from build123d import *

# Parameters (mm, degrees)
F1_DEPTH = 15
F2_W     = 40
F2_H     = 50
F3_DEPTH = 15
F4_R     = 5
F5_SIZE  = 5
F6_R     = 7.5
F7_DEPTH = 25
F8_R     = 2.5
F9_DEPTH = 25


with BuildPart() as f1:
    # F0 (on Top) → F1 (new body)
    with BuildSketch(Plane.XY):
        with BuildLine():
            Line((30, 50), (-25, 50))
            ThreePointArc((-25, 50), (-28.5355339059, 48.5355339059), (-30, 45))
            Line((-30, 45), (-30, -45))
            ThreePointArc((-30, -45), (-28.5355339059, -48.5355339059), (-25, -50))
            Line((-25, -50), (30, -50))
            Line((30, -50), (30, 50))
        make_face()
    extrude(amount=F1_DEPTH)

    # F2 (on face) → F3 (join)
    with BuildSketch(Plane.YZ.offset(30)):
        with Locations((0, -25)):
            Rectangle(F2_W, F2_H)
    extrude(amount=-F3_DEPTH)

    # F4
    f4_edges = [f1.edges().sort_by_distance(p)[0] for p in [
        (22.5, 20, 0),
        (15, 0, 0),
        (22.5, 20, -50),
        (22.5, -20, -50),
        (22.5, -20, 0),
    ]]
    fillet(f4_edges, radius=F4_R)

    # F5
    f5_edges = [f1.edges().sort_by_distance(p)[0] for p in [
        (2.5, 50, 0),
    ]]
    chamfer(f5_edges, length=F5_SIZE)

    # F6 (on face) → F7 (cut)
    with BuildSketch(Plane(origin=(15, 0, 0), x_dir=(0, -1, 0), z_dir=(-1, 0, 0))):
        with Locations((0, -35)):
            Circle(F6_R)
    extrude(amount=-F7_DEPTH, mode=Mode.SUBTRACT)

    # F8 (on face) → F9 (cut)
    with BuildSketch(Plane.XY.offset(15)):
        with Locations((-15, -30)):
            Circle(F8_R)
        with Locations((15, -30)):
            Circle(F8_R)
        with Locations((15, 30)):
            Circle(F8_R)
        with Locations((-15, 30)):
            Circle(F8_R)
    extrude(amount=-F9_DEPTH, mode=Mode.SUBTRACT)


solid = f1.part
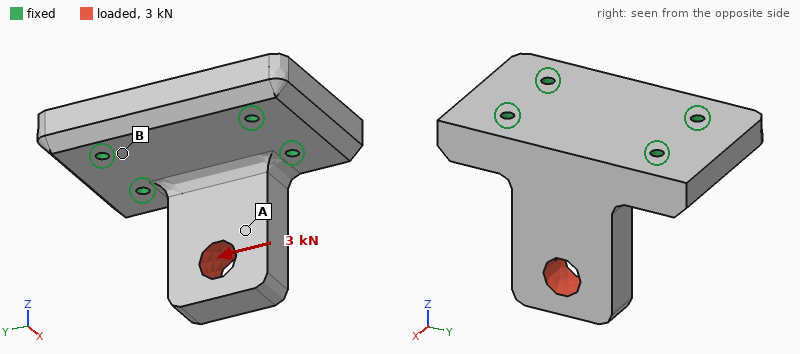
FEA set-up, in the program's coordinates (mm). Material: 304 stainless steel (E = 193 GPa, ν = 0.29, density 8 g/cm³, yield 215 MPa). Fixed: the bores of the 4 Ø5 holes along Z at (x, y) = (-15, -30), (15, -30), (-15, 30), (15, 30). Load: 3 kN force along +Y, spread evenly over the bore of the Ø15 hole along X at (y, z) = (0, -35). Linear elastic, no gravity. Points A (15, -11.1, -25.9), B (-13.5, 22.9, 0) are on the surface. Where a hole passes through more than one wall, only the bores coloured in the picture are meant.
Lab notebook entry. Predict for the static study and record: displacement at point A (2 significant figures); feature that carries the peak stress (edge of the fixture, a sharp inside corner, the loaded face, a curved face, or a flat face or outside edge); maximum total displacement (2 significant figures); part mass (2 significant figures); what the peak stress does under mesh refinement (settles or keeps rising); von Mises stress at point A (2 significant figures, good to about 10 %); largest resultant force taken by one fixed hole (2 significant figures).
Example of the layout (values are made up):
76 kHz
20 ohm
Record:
7.5 µm
a sharp inside corner
15 µm
910 g
keeps rising
8.5 MPa
2.7 kN
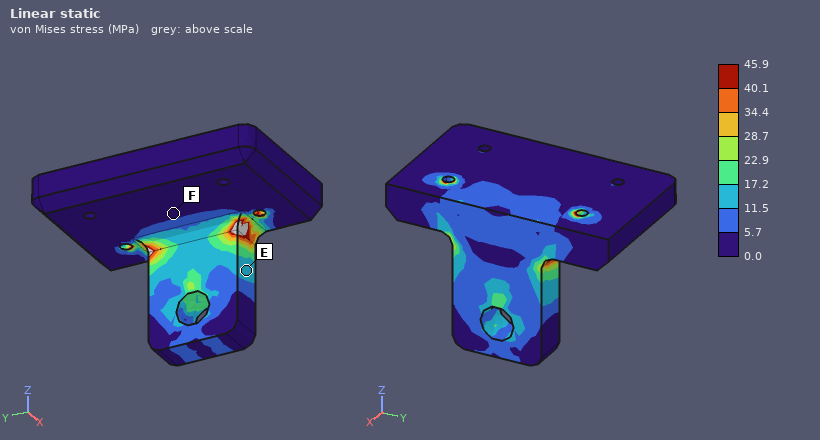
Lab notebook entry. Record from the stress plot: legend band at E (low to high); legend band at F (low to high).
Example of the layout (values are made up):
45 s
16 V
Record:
11.5 to 17.2 MPa
0.0 to 5.7 MPa
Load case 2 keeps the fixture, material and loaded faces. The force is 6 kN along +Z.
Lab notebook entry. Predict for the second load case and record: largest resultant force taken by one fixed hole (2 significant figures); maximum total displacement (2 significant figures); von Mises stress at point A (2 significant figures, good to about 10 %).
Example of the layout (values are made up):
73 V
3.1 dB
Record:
3.3 kN
14 µm
14 MPa
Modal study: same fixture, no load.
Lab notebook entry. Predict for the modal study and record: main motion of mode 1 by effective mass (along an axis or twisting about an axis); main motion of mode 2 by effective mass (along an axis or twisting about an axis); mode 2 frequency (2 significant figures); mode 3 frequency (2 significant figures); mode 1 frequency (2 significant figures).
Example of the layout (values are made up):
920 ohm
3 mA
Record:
along X
along Y
7000 Hz
9300 Hz
3400 Hz
